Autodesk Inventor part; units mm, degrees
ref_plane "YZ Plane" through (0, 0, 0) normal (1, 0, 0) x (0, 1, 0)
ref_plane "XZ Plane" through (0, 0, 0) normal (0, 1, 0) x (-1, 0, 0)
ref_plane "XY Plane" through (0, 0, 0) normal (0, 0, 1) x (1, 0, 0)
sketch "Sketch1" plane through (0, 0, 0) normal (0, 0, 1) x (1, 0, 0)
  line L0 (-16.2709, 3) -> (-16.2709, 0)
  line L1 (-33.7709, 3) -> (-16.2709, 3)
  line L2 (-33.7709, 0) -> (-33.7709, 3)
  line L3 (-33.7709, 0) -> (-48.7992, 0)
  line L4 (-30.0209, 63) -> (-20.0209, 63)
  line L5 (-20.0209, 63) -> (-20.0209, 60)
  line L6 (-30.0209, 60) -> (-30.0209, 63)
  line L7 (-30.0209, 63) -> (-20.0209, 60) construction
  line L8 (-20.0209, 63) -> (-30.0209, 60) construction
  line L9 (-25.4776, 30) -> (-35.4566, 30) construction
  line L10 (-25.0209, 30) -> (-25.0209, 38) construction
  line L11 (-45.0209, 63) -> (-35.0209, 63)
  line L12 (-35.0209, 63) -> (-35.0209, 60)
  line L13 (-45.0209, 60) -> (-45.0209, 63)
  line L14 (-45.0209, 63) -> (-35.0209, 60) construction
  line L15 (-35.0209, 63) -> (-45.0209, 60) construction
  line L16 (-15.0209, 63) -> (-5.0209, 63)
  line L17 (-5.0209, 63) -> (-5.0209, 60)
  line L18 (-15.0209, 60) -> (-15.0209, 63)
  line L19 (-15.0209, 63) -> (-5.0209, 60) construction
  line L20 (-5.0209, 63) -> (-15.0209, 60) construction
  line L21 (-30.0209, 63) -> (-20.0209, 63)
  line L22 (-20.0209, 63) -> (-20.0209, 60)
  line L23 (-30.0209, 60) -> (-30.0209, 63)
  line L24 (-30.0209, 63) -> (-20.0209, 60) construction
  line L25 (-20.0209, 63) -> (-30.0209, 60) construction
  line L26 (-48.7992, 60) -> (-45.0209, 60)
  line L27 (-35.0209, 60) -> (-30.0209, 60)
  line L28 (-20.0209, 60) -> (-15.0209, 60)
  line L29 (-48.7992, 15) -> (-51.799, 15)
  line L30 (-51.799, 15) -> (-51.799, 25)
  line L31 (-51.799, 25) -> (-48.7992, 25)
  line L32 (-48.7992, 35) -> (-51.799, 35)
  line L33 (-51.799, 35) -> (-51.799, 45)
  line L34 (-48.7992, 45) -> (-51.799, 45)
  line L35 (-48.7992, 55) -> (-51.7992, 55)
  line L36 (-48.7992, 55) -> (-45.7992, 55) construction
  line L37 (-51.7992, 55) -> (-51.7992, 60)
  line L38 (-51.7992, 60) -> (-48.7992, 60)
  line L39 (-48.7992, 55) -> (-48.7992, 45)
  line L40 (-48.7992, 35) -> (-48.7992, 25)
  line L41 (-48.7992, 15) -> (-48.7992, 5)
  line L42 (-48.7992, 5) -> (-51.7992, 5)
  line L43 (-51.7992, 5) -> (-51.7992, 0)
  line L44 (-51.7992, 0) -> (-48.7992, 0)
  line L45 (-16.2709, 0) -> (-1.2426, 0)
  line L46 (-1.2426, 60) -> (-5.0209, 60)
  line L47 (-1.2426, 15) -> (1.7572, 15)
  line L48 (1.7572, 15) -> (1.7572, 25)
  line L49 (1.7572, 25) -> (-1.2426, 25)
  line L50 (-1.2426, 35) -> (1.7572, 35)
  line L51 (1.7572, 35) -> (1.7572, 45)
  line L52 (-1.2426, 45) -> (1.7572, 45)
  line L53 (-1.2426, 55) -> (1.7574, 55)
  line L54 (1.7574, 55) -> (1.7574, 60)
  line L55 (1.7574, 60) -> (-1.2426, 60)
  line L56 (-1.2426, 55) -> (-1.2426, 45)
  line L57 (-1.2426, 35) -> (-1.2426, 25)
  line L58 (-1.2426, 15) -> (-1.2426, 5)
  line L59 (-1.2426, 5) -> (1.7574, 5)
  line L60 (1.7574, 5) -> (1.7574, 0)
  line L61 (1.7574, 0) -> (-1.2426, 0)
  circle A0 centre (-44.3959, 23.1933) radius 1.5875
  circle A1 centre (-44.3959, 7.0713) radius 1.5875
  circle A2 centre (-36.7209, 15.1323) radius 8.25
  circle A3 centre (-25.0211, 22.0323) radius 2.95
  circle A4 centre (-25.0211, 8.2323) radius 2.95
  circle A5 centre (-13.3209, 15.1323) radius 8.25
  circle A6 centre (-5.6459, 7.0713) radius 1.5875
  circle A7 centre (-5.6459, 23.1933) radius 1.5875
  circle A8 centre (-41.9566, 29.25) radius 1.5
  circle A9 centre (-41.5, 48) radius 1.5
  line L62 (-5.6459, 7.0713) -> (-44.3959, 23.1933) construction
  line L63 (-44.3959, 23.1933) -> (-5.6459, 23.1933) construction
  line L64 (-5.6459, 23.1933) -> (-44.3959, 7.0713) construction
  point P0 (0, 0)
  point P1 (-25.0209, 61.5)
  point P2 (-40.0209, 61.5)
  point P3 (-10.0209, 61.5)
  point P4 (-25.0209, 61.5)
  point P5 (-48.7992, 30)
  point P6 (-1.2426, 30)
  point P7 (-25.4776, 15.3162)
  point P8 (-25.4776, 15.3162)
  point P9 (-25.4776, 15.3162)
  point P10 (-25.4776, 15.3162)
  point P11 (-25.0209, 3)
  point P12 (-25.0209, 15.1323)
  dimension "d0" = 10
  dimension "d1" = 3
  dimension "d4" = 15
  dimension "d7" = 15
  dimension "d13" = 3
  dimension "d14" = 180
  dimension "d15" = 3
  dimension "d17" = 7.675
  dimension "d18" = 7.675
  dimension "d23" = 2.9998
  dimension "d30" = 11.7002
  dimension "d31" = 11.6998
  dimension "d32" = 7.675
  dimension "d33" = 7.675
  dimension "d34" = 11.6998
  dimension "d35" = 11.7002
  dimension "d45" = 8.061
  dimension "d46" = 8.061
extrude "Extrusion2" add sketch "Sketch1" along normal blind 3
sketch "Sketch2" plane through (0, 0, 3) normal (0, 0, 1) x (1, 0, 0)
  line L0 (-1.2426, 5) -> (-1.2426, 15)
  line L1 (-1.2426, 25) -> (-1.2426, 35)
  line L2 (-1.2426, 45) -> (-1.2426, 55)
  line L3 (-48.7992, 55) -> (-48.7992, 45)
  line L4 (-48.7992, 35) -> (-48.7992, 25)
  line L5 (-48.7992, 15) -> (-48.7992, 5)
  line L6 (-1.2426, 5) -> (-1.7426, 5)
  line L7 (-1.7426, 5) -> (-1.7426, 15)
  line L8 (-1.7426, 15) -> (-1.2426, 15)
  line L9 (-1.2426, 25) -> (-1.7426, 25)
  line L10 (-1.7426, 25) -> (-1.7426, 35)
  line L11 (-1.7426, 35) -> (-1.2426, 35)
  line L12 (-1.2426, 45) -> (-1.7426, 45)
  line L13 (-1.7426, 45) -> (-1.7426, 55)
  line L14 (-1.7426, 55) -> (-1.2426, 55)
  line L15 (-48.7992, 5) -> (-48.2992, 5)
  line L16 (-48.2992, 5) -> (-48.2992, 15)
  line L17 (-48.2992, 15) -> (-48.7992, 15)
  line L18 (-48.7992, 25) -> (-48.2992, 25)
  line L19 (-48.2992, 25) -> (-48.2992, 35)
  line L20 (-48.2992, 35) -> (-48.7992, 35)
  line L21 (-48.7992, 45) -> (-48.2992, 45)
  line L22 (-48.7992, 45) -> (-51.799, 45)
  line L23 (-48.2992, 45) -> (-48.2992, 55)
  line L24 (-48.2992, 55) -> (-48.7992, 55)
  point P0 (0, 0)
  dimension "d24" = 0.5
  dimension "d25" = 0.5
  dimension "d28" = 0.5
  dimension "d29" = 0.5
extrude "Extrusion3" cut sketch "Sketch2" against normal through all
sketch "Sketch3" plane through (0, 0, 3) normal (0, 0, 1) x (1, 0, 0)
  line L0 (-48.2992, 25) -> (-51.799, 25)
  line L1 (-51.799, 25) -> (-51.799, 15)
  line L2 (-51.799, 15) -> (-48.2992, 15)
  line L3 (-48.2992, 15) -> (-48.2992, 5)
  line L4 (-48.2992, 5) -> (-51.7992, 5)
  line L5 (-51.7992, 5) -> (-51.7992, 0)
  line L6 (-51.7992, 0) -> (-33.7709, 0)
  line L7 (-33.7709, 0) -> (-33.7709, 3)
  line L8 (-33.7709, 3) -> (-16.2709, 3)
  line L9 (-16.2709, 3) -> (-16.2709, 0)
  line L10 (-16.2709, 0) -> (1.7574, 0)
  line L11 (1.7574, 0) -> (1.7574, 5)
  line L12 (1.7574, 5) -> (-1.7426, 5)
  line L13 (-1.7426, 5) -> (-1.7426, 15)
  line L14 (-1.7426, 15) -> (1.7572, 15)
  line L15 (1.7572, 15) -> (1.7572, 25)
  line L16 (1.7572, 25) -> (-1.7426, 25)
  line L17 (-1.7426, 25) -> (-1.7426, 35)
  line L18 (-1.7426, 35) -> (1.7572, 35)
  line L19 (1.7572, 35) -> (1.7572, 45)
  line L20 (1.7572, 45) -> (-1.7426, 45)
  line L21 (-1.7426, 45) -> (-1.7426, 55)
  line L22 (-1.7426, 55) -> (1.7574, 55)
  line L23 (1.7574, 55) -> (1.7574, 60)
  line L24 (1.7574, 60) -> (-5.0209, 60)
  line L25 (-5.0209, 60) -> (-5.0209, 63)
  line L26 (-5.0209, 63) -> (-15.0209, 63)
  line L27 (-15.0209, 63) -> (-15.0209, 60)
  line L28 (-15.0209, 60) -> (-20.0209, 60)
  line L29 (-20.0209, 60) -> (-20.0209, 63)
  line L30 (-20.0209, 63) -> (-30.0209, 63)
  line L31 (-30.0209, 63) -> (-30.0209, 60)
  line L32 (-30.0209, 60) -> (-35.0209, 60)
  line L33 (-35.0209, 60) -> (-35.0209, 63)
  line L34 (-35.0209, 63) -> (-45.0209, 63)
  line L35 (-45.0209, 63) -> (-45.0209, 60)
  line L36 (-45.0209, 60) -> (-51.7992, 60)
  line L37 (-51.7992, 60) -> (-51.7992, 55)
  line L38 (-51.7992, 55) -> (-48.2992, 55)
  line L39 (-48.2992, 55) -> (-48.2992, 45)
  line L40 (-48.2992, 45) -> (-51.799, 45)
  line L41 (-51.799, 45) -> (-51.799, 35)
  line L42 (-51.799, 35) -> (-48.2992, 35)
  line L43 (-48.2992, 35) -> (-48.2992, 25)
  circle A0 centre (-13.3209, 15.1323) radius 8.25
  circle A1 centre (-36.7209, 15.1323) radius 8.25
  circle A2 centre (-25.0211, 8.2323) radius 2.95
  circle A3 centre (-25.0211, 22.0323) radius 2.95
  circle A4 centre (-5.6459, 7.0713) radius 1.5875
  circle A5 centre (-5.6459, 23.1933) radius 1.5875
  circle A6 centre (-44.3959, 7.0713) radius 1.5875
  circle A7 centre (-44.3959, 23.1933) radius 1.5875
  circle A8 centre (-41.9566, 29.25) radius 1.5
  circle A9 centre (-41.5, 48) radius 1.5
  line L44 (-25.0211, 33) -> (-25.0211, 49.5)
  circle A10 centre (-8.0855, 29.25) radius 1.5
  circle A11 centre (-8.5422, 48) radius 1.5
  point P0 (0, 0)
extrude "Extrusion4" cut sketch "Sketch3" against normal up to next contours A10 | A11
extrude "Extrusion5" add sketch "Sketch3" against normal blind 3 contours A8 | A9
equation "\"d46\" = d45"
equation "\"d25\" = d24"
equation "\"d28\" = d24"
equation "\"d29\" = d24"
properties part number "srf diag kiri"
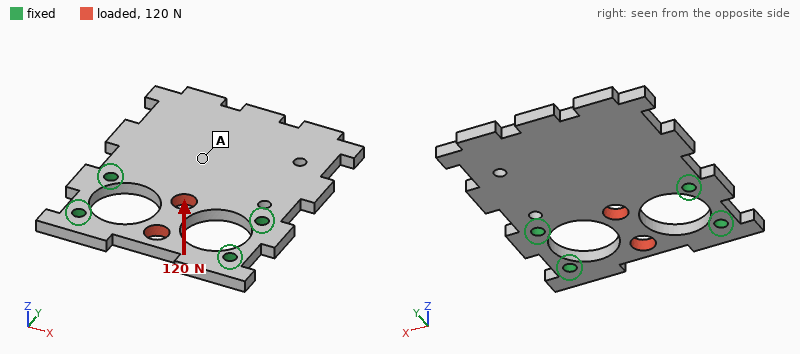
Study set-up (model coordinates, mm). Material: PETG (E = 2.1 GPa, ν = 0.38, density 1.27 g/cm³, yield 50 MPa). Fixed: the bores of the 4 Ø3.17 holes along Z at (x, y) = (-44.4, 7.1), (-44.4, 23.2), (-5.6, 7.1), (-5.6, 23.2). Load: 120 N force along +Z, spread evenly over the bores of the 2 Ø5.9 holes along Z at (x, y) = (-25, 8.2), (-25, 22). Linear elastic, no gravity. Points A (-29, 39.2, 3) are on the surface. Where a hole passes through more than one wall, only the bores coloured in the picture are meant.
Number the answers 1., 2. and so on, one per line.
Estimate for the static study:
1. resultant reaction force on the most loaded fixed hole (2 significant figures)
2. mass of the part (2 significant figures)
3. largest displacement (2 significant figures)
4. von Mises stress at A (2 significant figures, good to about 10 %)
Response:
1. 31 N
2. 9.6 g
3. 0.65 mm
4. 3.4 MPa
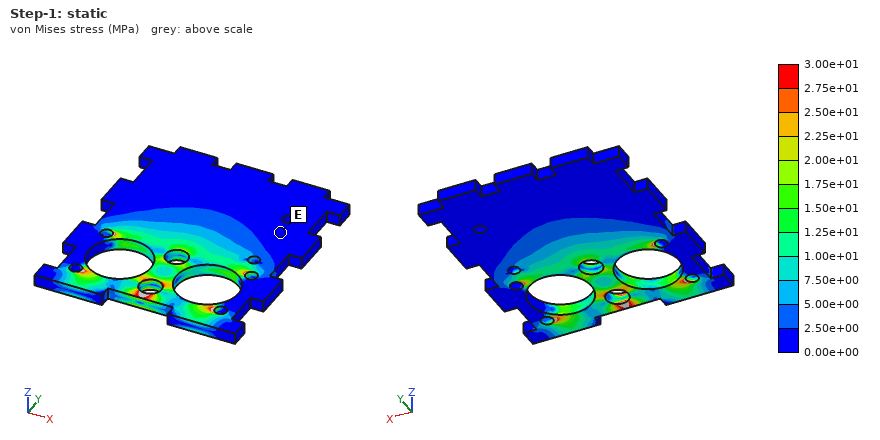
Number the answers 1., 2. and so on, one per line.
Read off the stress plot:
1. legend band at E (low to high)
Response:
1. 0.00e+00 to 2.50e+00 MPa
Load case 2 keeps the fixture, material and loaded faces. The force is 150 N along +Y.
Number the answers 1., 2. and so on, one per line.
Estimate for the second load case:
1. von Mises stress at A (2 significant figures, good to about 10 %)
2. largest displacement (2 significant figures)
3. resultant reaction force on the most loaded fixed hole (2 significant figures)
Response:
1. 1.2 MPa
2. 87 µm
3. 63 N
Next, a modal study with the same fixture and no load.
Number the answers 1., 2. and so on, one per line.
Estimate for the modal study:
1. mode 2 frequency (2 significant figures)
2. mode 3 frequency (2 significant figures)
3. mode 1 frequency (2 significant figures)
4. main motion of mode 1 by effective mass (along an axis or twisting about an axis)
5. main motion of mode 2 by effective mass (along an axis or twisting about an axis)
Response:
1. 790 Hz
2. 1900 Hz
3. 330 Hz
4. along Z
5. twisting about Y
